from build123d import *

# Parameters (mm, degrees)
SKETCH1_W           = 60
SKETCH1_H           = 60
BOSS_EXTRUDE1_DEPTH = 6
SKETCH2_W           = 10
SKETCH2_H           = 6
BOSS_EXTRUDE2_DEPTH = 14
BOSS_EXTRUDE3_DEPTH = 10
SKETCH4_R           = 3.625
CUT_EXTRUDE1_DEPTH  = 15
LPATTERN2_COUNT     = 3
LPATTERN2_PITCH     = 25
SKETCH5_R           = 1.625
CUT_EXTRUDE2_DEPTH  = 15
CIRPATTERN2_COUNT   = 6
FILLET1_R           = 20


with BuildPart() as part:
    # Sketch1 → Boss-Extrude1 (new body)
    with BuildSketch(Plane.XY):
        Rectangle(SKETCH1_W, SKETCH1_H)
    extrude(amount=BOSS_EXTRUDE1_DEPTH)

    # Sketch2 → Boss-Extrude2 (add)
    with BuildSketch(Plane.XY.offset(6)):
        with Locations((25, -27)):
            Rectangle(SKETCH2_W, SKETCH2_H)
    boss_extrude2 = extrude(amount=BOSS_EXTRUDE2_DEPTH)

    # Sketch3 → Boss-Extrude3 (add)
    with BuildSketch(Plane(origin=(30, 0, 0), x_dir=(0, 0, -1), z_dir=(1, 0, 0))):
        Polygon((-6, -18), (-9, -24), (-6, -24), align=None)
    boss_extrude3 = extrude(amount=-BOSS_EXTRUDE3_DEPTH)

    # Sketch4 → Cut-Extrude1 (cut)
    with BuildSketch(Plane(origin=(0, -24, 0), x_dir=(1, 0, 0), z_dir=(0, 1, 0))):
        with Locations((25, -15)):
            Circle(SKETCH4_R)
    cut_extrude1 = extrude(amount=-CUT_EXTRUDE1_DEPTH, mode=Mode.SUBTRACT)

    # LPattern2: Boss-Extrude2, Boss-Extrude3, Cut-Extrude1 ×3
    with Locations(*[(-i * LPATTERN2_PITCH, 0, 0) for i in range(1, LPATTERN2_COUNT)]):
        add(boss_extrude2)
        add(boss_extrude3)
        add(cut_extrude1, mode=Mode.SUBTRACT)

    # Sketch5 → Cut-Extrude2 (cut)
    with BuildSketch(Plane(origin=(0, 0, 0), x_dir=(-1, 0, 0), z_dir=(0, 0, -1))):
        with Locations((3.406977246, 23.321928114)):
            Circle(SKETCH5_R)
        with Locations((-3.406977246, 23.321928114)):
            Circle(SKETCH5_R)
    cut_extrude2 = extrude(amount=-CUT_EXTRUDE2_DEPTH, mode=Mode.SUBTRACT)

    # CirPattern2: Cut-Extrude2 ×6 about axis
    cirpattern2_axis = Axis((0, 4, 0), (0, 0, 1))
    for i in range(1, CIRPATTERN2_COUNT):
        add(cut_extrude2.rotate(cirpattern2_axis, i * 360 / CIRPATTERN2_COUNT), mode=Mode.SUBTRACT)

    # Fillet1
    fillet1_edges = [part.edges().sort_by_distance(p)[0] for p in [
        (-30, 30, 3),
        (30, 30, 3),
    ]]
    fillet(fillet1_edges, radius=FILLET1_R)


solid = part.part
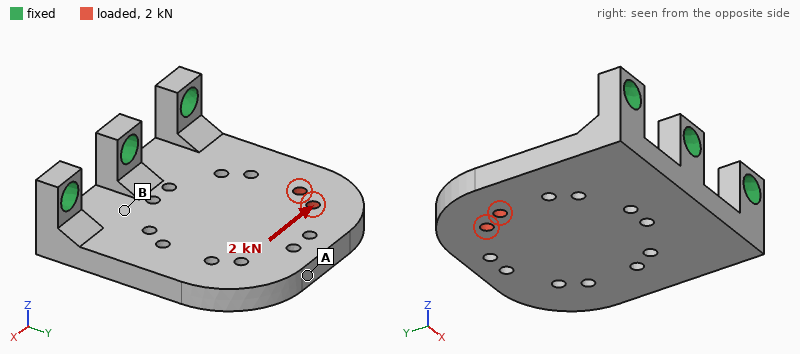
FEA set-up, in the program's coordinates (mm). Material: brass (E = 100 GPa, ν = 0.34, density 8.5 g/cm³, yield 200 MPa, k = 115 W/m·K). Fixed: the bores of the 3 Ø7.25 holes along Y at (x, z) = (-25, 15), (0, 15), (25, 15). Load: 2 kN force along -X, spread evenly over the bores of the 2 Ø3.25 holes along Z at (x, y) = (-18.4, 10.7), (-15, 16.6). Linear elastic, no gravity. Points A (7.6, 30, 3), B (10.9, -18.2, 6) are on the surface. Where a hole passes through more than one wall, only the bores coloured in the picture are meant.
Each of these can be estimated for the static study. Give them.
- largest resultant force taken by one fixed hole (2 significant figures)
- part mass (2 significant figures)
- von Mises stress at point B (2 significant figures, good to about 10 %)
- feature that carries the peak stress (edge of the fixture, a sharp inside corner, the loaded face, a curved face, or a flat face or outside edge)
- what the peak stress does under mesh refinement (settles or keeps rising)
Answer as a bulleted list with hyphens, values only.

- 1.7 kN
- 190 g
- 28 MPa
- edge of the fixture
- keeps rising
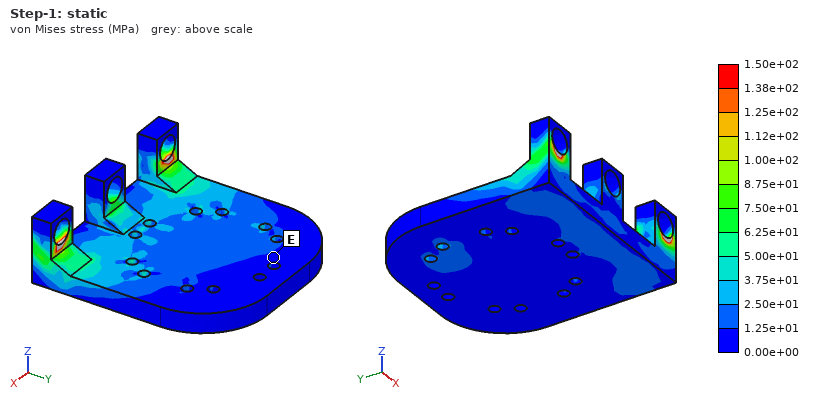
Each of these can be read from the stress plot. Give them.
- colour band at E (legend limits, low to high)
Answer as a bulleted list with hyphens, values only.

- 0.00e+00 to 1.25e+01 MPa
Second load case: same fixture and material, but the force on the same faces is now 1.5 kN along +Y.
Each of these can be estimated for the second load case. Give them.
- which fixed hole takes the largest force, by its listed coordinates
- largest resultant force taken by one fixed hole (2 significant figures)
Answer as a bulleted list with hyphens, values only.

- (-25, 15)
- 970 N
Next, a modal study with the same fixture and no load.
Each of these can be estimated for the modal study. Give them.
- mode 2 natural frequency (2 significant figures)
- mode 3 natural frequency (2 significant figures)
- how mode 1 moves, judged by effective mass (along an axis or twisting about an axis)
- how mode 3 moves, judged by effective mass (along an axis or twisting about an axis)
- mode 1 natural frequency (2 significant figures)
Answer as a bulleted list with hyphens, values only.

- 2400 Hz
- 4000 Hz
- along Z
- along X
- 870 Hz
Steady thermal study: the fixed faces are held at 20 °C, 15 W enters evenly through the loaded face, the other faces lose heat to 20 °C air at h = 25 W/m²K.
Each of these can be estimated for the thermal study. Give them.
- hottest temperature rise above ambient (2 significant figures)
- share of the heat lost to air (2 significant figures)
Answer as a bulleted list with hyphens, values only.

- 25 K
- 16 %
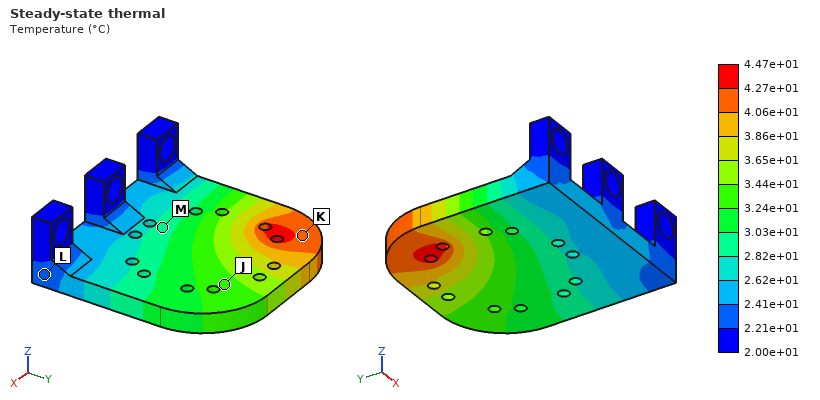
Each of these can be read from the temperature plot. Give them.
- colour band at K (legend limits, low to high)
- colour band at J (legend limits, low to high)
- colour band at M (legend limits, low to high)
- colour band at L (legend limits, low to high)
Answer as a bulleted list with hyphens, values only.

- 4.06e+01 to 4.27e+01 °C
- 3.24e+01 to 3.44e+01 °C
- 2.82e+01 to 3.03e+01 °C
- 2.21e+01 to 2.41e+01 °C
